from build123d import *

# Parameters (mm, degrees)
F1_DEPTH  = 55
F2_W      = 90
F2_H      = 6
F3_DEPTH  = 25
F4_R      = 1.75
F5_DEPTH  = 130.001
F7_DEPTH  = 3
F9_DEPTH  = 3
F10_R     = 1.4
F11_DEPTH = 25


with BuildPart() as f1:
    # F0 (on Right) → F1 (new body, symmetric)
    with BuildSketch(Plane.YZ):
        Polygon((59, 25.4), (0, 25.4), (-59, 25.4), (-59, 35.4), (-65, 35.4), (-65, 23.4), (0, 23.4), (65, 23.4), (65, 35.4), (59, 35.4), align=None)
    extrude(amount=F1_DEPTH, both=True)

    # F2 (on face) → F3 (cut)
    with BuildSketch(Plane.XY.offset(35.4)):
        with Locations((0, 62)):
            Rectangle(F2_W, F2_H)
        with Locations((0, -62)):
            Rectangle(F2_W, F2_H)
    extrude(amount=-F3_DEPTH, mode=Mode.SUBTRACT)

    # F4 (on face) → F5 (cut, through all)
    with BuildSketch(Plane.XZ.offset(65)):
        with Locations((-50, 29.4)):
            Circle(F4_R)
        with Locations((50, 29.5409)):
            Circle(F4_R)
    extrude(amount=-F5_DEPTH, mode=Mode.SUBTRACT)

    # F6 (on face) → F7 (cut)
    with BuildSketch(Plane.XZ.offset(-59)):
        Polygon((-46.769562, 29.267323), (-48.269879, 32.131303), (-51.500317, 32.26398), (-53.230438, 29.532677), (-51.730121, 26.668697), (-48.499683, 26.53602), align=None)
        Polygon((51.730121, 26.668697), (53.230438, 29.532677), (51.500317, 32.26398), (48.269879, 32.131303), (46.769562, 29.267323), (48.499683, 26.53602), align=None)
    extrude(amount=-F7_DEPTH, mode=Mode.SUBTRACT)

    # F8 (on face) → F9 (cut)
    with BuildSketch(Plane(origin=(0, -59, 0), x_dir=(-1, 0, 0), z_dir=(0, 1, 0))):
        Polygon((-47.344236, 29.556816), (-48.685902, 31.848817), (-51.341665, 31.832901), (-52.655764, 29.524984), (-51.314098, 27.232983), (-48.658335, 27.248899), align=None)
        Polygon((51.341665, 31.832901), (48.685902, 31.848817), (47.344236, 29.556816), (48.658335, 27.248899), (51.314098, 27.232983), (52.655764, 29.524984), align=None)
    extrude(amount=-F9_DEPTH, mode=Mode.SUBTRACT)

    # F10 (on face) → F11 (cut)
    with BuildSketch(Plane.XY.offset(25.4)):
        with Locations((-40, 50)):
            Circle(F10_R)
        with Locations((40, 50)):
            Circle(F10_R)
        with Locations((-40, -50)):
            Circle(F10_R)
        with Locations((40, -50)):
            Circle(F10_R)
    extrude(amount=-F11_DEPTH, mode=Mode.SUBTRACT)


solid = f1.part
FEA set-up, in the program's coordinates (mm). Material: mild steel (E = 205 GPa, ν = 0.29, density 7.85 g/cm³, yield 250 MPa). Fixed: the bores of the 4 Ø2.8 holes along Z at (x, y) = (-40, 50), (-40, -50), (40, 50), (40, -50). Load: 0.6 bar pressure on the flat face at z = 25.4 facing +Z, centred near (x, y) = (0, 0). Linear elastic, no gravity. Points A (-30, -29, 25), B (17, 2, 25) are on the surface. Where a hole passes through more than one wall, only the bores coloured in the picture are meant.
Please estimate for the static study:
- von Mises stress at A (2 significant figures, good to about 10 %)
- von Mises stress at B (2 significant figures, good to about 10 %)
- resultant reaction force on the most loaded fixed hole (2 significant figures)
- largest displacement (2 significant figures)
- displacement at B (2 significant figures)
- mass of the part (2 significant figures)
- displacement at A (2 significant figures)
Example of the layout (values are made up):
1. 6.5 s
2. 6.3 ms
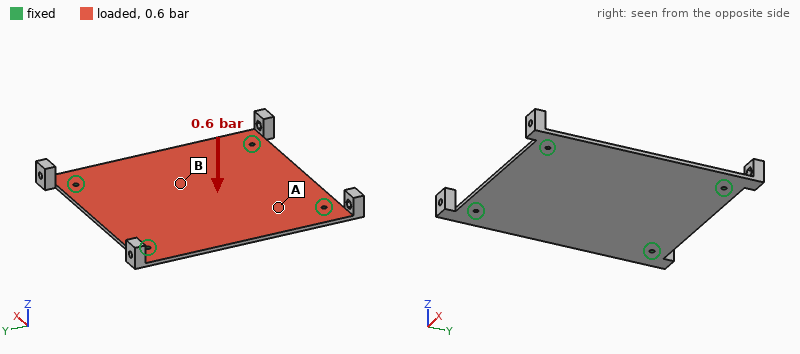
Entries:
1. 17 MPa
2. 41 MPa
3. 190 N
4. 0.22 mm
5. 0.21 mm
6. 220 g
7. 0.11 mm
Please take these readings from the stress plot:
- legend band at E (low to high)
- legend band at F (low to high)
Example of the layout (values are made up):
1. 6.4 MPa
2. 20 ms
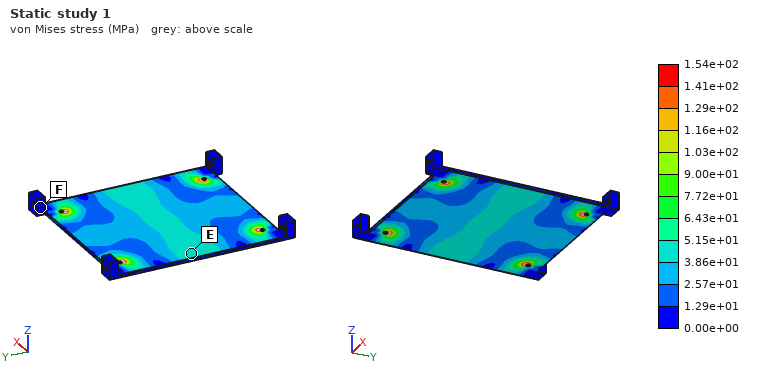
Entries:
1. 3.86e+01 to 5.15e+01 MPa
2. 0.00e+00 to 1.29e+01 MPa
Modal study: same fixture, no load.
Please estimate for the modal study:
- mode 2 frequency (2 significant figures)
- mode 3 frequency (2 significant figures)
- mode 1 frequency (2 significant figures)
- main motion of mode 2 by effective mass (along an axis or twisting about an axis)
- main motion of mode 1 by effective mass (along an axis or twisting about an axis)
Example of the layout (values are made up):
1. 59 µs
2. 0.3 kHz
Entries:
1. 1100 Hz
2. 1400 Hz
3. 790 Hz
4. twisting about Y
5. along Z
